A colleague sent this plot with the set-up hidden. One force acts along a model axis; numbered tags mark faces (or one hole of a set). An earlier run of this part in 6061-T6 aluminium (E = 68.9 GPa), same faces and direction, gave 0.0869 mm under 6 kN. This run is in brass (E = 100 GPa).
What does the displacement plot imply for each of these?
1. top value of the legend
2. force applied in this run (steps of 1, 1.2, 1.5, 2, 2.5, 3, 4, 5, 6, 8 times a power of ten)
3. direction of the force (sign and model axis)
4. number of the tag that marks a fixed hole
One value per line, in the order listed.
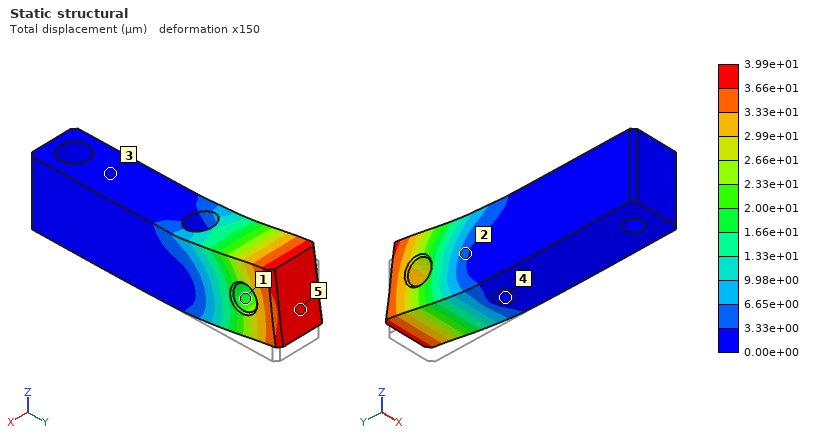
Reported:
3.99e+01 µm
4 kN
+Z
4
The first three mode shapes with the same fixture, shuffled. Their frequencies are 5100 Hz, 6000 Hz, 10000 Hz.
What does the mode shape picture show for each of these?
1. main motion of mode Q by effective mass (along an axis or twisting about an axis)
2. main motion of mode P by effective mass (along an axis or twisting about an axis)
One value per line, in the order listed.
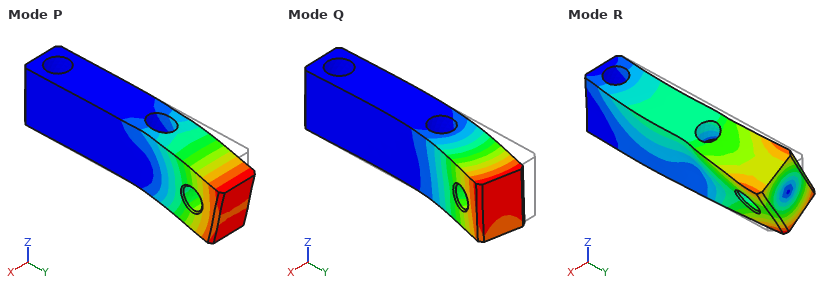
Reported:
along X
along Z
